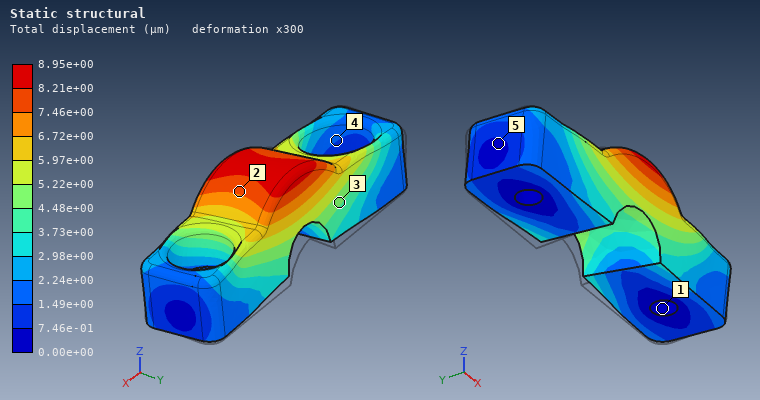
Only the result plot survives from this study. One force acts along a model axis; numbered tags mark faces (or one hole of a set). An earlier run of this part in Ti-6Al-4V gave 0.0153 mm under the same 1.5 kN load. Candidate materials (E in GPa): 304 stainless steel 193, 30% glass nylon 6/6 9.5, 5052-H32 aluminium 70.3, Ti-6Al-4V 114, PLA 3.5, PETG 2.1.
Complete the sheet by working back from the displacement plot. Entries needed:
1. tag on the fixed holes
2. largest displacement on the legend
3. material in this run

1
8.95e+00 µm
304 stainless steel
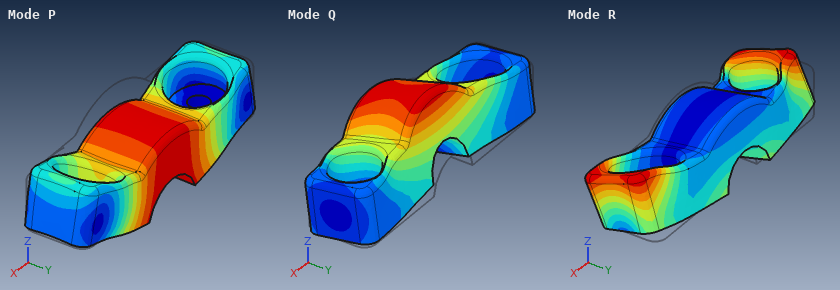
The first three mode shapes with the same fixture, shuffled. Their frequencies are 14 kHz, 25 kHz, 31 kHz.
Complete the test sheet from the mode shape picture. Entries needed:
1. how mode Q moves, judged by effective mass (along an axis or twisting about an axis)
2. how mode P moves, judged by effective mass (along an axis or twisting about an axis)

along Y
along Z
